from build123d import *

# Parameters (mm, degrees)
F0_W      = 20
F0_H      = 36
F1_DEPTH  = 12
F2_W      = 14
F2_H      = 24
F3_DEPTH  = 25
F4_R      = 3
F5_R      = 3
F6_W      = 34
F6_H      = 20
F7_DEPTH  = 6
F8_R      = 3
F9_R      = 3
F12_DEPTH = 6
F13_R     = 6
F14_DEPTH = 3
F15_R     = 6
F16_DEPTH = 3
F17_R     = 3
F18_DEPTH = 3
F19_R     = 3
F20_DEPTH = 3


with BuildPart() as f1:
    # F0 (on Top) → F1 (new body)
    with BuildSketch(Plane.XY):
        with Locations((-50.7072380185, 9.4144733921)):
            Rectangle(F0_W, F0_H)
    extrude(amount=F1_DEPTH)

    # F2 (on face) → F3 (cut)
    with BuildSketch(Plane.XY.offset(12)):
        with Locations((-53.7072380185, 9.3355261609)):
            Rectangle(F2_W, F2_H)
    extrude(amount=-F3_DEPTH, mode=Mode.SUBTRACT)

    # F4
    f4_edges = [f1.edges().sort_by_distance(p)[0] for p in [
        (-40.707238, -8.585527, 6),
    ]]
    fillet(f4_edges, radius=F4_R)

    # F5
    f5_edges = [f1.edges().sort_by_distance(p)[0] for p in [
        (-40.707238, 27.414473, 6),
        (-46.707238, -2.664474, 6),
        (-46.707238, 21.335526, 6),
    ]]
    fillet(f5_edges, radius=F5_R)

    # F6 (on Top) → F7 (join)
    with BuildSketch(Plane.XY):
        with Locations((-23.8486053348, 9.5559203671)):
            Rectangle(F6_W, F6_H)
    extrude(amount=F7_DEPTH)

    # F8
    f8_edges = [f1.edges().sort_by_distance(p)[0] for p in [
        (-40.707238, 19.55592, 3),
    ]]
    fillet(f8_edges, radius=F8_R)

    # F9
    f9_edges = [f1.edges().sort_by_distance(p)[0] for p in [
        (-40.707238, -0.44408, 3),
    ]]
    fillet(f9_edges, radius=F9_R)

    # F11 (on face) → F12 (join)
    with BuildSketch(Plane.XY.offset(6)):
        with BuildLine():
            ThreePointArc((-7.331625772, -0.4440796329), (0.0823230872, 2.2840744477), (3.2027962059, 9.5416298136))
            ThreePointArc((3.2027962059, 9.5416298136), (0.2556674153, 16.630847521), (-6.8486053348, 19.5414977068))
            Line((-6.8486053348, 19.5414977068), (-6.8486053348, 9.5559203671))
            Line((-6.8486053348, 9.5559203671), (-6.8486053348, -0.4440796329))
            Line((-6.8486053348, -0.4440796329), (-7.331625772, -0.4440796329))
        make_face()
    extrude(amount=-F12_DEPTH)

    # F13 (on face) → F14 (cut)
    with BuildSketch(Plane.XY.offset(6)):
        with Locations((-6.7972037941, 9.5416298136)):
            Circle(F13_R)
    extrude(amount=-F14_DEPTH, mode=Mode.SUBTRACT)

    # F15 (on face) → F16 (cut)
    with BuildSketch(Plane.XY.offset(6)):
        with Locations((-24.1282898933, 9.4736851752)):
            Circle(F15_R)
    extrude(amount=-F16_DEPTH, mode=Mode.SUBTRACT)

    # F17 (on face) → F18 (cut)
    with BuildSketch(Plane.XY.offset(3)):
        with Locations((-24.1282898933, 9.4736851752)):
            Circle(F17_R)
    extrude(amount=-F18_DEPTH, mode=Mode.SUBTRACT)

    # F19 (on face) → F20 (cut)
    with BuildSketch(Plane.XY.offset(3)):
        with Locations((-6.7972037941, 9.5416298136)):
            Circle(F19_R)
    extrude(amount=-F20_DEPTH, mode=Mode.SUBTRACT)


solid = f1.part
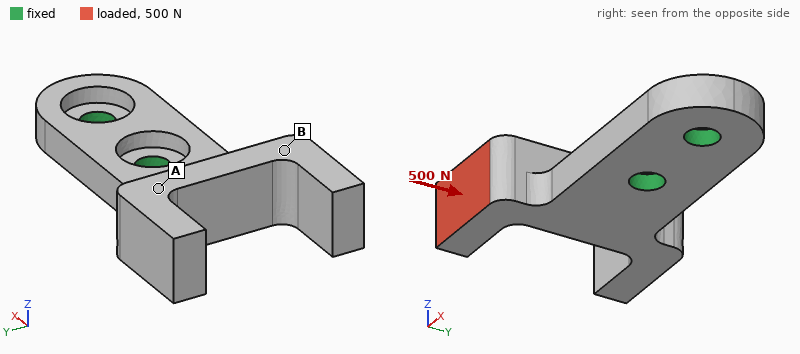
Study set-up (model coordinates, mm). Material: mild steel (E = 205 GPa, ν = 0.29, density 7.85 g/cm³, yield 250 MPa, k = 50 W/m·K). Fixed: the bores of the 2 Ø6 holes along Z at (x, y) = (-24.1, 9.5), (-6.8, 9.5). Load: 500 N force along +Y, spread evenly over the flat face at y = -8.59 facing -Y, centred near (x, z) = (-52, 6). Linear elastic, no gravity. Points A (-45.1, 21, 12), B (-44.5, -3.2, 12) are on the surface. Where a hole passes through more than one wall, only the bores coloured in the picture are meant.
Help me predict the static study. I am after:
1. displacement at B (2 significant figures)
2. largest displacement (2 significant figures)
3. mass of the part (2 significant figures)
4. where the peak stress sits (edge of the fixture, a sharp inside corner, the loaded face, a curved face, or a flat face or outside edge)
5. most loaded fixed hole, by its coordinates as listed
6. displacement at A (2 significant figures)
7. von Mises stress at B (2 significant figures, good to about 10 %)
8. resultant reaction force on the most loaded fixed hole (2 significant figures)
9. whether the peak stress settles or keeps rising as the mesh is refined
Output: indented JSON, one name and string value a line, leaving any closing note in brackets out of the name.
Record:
{
  "displacement at B": "15 µm",
  "largest displacement": "36 µm",
  "mass of the part": "69 g",
  "where the peak stress sits": "edge of the fixture",
  "most loaded fixed hole, by its coordinates as listed": "(-24.1, 9.5)",
  "displacement at A": "13 µm",
  "von Mises stress at B": "18 MPa",
  "resultant reaction force on the most loaded fixed hole": "950 N",
  "whether the peak stress settles or keeps rising as the mesh is refined": "keeps rising"
}
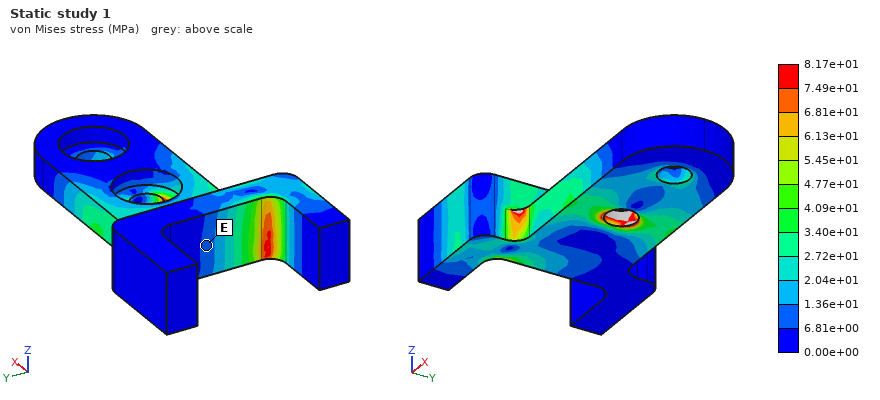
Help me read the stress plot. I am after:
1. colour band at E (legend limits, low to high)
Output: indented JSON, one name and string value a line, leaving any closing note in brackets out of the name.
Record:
{
  "colour band at E": "6.81e+00 to 1.36e+01 MPa"
}
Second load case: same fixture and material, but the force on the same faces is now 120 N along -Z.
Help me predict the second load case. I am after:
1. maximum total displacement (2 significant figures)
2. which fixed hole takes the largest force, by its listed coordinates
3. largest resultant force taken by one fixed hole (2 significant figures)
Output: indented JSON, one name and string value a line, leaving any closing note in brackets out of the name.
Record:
{
  "maximum total displacement": "41 µm",
  "which fixed hole takes the largest force, by its listed coordinates": "(-24.1, 9.5)",
  "largest resultant force taken by one fixed hole": "290 N"
}
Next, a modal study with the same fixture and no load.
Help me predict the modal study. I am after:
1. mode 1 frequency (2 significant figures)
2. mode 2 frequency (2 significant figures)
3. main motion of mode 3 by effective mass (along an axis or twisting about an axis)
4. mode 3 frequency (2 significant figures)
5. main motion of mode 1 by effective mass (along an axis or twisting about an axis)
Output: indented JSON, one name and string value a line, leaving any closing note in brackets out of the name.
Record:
{
  "mode 1 frequency": "2400 Hz",
  "mode 2 frequency": "3500 Hz",
  "main motion of mode 3 by effective mass": "along Y",
  "mode 3 frequency": "5200 Hz",
  "main motion of mode 1 by effective mass": "along Z"
}
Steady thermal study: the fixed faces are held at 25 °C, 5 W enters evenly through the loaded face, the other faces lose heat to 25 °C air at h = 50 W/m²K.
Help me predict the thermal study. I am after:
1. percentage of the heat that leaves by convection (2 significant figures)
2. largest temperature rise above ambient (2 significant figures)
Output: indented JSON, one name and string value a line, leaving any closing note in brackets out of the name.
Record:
{
  "percentage of the heat that leaves by convection": "37 %",
  "largest temperature rise above ambient": "31 K"
}
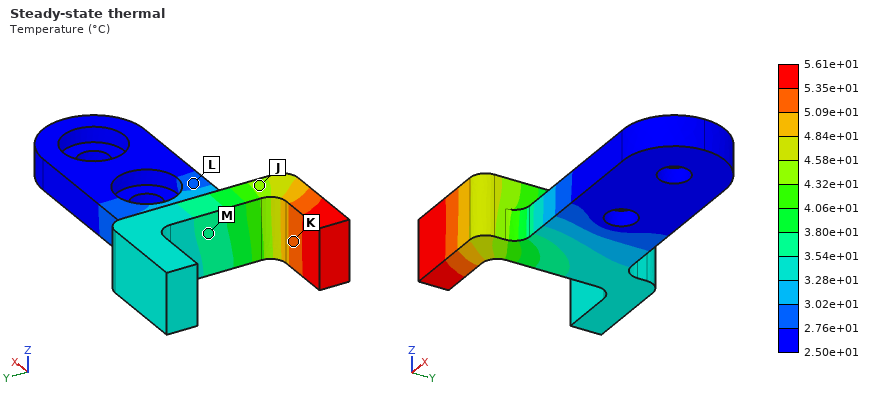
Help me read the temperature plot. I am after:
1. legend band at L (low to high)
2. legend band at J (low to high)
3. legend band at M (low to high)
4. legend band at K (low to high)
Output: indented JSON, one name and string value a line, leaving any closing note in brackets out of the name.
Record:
{
  "legend band at L": "2.76e+01 to 3.02e+01 °C",
  "legend band at J": "4.32e+01 to 4.58e+01 °C",
  "legend band at M": "3.54e+01 to 3.80e+01 °C",
  "legend band at K": "5.09e+01 to 5.35e+01 °C"
}
